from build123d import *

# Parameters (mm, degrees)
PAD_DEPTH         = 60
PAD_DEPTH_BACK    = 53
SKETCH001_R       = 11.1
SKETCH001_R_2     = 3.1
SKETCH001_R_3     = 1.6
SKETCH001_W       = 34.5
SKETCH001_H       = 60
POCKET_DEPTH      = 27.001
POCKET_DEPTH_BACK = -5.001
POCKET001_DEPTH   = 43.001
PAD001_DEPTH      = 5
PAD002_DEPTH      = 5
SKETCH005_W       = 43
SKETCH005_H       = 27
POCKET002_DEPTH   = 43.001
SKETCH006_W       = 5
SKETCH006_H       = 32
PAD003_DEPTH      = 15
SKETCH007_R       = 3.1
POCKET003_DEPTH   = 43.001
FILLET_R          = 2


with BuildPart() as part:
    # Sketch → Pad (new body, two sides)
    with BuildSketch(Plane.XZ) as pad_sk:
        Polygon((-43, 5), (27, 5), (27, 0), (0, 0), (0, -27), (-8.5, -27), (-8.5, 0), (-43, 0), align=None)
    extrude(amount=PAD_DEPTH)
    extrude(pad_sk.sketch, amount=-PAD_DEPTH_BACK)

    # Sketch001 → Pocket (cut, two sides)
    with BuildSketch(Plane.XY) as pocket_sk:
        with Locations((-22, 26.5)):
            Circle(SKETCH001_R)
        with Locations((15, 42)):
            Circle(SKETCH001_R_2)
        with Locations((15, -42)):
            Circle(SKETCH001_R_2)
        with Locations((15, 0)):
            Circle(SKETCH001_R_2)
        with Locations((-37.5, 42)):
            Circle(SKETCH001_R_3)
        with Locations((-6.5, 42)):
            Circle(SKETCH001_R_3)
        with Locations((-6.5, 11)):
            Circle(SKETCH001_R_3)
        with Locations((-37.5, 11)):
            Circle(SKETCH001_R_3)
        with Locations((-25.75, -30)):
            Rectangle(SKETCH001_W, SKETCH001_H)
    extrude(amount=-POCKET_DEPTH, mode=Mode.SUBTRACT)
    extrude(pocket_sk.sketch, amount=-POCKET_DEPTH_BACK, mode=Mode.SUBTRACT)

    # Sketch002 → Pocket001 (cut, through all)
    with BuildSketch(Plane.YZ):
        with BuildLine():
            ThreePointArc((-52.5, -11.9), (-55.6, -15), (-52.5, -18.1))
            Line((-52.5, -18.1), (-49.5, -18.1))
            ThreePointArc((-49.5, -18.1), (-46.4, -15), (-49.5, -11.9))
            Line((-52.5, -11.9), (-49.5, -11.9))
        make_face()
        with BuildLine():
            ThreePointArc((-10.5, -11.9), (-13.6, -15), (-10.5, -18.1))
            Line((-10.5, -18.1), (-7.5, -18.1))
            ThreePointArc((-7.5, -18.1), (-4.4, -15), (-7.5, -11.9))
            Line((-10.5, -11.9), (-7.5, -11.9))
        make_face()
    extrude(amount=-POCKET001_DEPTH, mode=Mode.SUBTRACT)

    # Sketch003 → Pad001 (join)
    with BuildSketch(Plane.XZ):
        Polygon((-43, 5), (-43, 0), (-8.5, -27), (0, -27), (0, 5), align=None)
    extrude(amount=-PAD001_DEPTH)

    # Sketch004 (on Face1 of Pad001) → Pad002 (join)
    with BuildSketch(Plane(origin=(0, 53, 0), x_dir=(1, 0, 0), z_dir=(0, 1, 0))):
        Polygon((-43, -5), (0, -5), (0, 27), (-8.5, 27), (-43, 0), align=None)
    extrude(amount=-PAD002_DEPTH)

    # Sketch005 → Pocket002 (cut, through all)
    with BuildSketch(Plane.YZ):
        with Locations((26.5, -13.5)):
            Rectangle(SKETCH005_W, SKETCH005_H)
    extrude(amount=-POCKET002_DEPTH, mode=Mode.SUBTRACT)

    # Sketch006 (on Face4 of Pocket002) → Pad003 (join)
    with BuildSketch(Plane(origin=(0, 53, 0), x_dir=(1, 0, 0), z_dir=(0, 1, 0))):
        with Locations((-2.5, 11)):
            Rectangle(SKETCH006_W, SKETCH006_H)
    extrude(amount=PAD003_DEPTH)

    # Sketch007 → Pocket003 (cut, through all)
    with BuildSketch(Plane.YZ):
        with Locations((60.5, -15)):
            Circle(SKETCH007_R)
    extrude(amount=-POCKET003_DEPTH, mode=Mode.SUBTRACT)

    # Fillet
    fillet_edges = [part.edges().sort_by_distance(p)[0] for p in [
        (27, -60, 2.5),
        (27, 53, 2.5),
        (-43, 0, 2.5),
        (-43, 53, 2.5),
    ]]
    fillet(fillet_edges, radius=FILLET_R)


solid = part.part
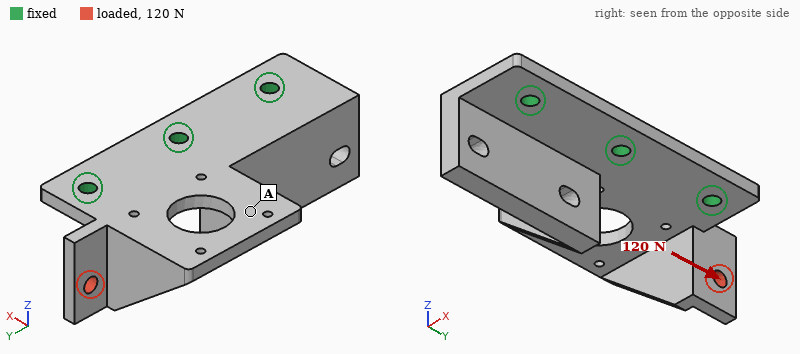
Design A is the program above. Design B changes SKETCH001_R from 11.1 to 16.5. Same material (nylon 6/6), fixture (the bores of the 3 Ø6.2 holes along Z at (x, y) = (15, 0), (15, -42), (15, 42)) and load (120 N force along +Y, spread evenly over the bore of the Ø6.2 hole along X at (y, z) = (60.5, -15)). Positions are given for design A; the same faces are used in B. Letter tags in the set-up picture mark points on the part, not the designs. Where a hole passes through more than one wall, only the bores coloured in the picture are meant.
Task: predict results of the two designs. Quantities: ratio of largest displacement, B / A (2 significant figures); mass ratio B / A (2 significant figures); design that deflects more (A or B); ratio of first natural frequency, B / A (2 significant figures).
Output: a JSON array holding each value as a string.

["1.2", "0.95", "B", "1.0"]
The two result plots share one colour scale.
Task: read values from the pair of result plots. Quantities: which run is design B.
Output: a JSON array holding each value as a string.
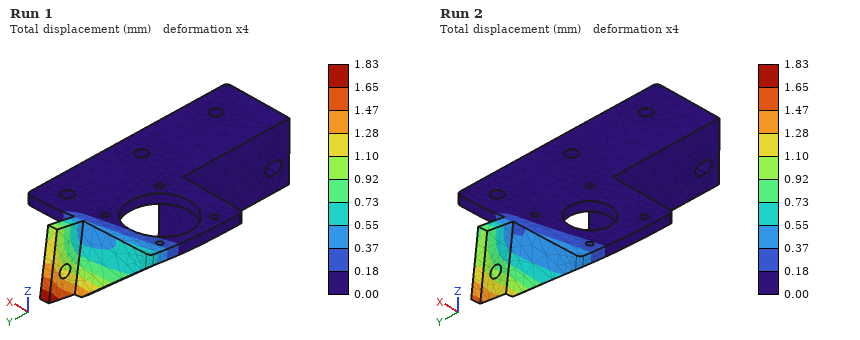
["Run 1"]
